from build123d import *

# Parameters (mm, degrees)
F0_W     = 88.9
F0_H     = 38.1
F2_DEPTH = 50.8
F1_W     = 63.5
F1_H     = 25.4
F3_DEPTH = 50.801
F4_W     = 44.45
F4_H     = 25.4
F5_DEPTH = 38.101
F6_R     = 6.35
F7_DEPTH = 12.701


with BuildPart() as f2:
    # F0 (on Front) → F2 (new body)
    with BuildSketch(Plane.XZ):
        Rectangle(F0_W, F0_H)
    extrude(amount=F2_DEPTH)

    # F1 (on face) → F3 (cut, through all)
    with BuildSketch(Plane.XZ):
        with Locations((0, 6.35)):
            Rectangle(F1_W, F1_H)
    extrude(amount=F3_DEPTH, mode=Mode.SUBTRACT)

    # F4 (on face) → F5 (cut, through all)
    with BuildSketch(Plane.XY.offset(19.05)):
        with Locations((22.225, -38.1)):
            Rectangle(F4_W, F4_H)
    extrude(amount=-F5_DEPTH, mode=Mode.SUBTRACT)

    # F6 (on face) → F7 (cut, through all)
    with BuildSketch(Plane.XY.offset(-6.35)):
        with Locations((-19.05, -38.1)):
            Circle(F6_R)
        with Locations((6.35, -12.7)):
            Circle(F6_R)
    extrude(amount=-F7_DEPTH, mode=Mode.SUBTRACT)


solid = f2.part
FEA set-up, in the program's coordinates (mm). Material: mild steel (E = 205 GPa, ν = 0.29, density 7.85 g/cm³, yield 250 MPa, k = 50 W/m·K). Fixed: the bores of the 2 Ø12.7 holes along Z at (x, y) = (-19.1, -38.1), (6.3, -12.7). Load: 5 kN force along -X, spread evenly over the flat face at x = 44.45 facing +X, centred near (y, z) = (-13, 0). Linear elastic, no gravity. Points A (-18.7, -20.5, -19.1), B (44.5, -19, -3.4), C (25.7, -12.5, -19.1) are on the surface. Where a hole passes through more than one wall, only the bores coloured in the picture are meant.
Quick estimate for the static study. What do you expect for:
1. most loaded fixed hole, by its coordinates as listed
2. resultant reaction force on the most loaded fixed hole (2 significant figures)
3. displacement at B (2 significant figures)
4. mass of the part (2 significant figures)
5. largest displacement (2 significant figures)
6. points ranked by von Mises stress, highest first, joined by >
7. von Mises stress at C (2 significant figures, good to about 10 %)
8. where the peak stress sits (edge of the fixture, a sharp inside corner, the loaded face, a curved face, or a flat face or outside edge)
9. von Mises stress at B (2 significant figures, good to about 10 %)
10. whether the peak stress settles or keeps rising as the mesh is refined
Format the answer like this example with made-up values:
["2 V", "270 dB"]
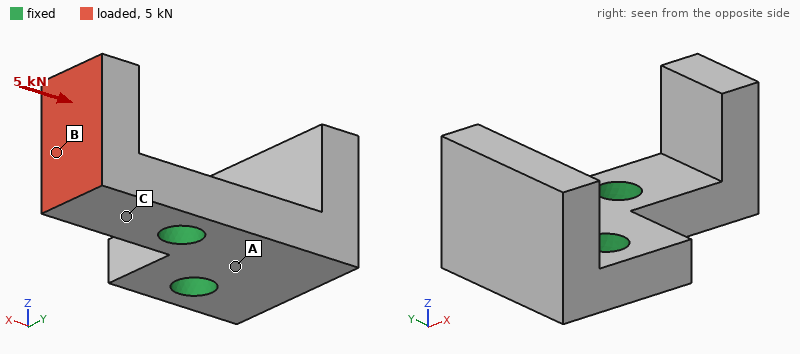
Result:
["(6.3, -12.7)", "4.9 kN", "46 µm", "510 g", "86 µm", "C > B > A", "73 MPa", "edge of the fixture", "50 MPa", "keeps rising"]
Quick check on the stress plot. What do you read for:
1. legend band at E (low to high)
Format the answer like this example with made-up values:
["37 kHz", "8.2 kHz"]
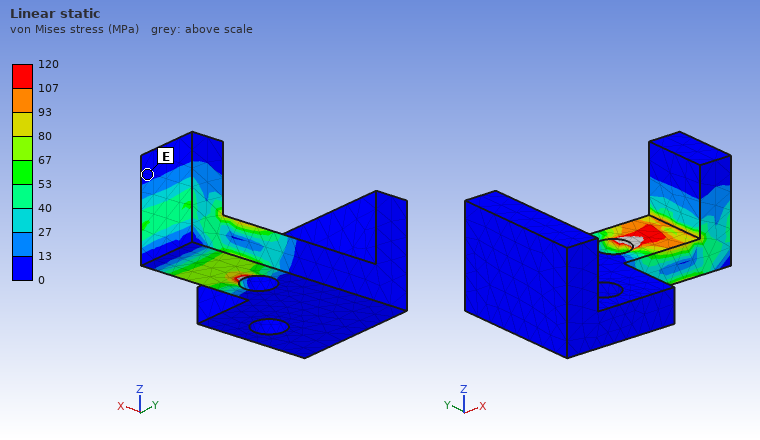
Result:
["0 to 13 MPa"]
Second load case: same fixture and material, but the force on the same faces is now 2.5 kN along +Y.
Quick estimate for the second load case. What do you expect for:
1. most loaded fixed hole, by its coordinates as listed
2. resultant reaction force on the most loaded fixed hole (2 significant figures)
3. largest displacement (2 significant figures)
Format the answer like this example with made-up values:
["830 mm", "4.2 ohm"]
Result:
["(6.3, -12.7)", "2.9 kN", "43 µm"]
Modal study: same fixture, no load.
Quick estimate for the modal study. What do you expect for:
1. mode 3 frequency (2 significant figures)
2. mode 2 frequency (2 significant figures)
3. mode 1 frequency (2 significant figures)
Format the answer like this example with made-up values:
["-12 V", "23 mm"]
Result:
["4800 Hz", "4700 Hz", "3800 Hz"]
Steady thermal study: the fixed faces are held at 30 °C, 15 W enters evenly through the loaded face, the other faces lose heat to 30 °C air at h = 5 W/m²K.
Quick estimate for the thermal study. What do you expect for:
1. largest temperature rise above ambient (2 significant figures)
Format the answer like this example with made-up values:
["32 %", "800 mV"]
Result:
["34 K"]
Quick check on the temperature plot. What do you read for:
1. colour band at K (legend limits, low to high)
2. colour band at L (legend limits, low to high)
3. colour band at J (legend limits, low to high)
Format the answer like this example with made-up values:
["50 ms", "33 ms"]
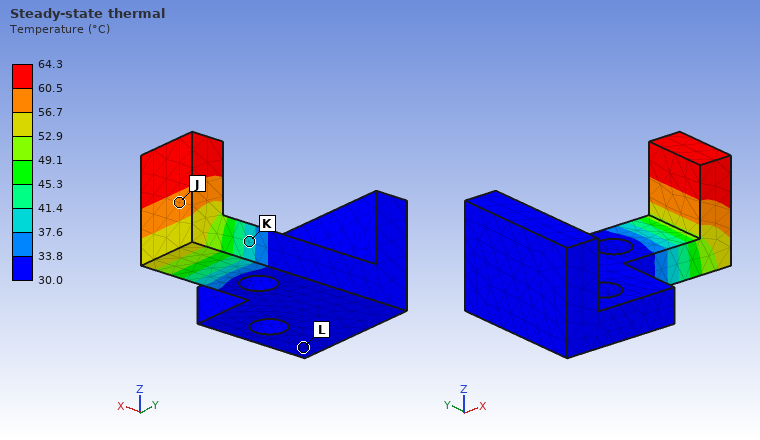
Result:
["37.6 to 41.4 °C", "30.0 to 33.8 °C", "56.7 to 60.5 °C"]
